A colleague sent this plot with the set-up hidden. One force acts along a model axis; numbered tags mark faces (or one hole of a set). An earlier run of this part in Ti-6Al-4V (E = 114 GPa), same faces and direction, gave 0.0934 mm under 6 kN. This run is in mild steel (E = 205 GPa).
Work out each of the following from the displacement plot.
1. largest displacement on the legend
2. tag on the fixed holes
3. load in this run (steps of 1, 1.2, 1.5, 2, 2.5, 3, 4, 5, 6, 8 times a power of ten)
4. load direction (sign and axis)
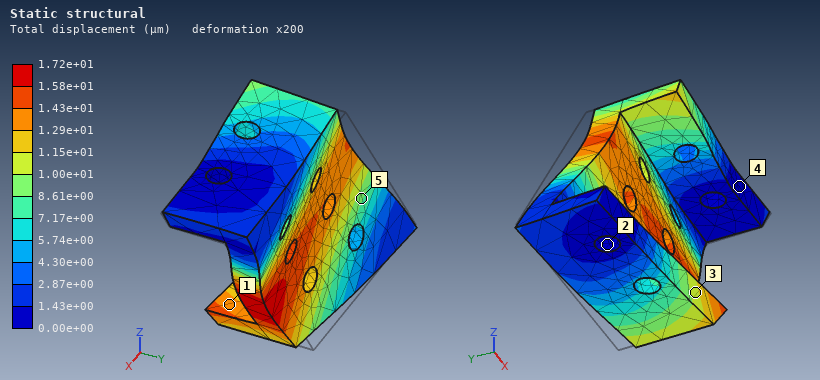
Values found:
1.72e+01 µm
2
2 kN
-Y
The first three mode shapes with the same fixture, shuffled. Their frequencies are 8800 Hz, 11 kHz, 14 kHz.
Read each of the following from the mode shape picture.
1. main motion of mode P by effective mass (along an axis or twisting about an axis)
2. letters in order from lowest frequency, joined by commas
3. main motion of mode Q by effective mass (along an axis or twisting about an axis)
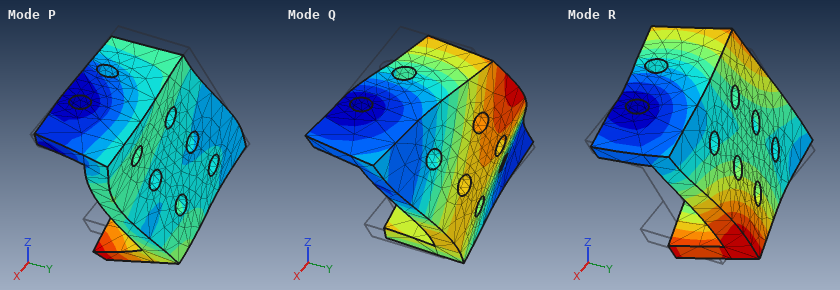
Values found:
along Z
R, Q, P
along Y
